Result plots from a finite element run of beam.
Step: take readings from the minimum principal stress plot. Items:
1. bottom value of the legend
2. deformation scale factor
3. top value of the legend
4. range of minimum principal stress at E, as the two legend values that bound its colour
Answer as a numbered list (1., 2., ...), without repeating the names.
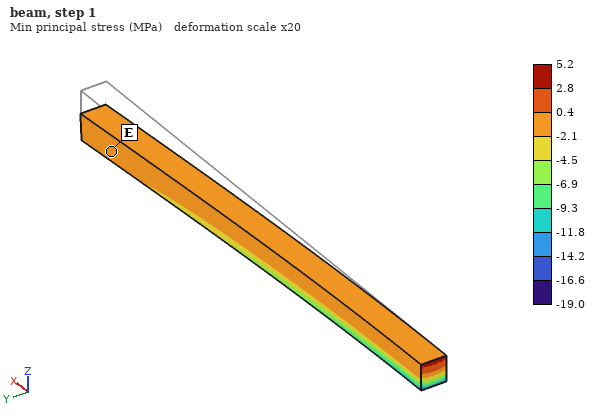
1. -19.0 MPa
2. 20
3. 5.2 MPa
4. -2.1 to 0.4 MPa
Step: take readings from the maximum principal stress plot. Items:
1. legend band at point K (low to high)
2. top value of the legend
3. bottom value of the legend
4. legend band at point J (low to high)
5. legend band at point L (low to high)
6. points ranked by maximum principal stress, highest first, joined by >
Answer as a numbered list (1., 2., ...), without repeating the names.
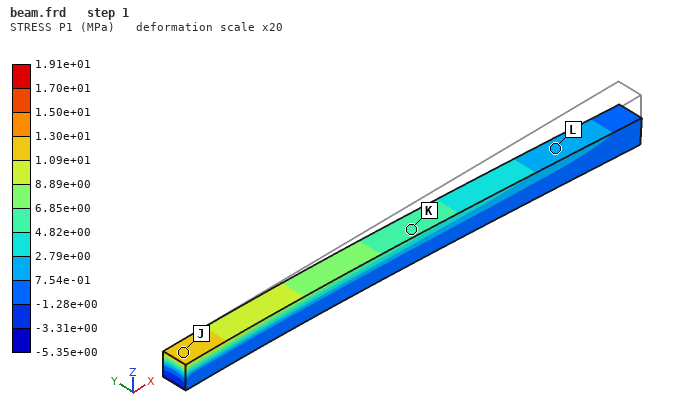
1. 4.82e+00 to 6.85e+00 MPa
2. 1.91e+01 MPa
3. -5.35e+00 MPa
4. 1.09e+01 to 1.30e+01 MPa
5. 7.54e-01 to 2.79e+00 MPa
6. J > K > L
